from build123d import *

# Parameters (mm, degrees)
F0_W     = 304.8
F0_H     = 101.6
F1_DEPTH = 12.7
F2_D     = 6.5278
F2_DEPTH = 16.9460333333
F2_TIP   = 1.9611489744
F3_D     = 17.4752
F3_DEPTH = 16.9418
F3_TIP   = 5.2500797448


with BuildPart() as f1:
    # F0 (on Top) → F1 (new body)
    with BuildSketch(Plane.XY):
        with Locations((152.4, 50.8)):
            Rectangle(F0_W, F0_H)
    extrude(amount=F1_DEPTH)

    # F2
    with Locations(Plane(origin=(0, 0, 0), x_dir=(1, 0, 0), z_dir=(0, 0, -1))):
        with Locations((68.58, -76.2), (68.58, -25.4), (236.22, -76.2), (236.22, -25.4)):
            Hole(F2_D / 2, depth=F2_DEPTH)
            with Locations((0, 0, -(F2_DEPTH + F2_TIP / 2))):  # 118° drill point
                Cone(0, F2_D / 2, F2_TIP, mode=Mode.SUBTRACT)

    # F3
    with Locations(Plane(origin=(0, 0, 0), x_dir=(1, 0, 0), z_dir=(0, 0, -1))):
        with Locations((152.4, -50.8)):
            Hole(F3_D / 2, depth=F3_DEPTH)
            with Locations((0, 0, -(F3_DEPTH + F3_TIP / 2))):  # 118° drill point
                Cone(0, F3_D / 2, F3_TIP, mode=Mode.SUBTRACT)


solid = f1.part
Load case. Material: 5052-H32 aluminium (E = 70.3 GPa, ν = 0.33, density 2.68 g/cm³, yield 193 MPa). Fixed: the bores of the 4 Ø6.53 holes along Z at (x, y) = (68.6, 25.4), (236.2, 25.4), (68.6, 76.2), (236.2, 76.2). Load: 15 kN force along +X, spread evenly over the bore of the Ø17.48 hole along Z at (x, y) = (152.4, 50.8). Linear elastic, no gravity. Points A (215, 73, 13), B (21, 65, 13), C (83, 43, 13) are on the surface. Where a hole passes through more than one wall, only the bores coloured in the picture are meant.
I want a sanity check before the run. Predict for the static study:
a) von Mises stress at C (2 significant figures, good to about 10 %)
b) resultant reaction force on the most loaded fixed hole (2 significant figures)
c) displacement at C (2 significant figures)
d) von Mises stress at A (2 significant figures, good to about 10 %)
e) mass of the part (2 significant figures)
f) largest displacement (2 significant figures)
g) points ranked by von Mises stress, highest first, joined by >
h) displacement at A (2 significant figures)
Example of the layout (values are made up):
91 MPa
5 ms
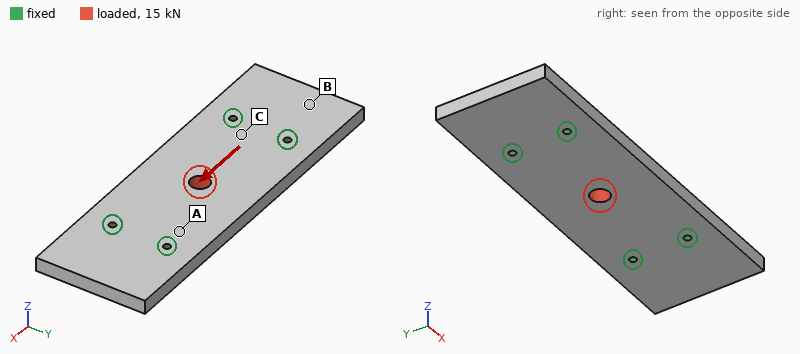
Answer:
5.4 MPa
3.8 kN
2.8 µm
8.5 MPa
1.0 kg
13 µm
A > C > B
3.0 µm
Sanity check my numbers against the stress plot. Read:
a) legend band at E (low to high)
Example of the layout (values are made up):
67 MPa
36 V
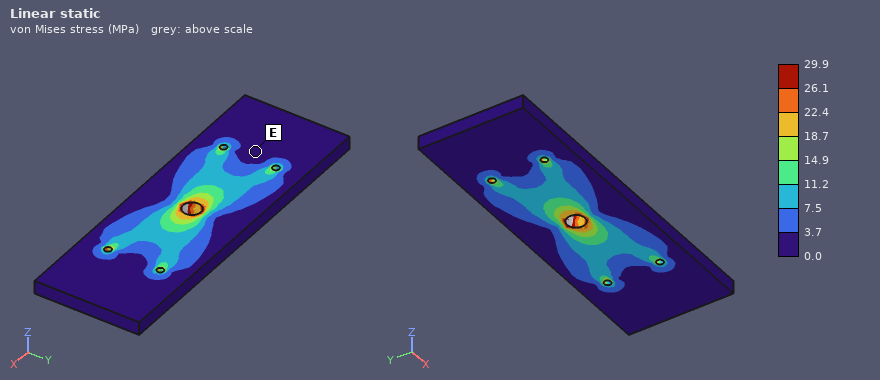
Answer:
0.0 to 3.7 MPa
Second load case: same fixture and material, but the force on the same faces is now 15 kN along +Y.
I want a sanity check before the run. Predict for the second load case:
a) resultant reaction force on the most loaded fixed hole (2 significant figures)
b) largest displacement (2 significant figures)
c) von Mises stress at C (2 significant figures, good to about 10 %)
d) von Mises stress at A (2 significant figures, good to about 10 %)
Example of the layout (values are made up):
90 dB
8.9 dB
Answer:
5.7 kN
33 µm
15 MPa
13 MPa
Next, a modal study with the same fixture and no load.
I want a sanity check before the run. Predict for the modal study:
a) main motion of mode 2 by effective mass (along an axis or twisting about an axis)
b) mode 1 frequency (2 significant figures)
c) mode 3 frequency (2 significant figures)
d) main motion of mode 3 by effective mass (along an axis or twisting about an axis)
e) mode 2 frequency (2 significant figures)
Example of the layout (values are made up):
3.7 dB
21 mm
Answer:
twisting about Y
1800 Hz
2300 Hz
along Z
2000 Hz
